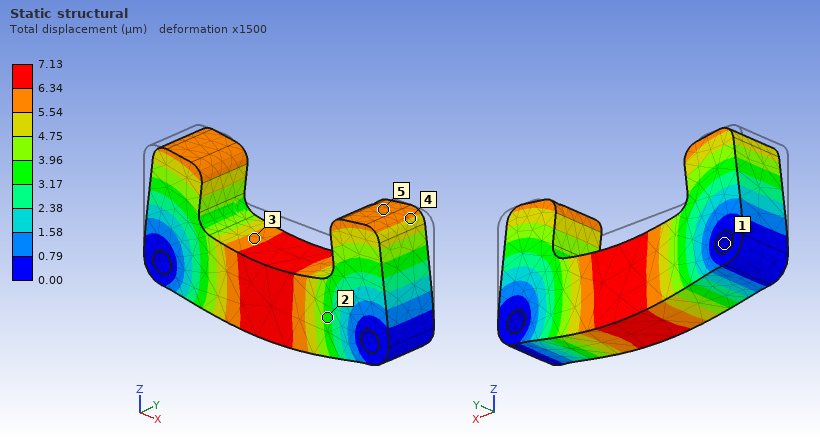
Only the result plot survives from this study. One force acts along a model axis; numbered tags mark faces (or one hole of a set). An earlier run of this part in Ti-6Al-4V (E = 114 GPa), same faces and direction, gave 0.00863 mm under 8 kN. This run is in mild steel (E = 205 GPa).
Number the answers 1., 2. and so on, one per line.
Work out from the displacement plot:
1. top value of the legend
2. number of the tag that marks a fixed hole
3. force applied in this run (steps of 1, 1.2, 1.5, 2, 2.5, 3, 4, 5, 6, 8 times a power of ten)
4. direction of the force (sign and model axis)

1. 7.13 µm
2. 1
3. 12 kN
4. -Z
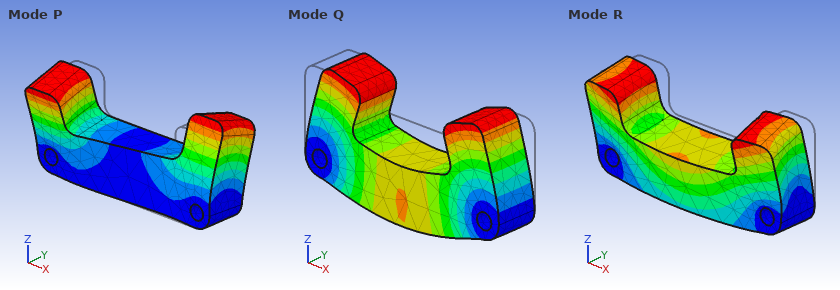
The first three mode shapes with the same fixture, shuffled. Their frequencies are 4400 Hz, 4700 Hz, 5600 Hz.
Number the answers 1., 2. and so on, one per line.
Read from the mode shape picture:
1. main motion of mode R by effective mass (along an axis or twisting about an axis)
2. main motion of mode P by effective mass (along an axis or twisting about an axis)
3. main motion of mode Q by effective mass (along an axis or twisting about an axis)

1. along Y
2. twisting about Z
3. along Z
